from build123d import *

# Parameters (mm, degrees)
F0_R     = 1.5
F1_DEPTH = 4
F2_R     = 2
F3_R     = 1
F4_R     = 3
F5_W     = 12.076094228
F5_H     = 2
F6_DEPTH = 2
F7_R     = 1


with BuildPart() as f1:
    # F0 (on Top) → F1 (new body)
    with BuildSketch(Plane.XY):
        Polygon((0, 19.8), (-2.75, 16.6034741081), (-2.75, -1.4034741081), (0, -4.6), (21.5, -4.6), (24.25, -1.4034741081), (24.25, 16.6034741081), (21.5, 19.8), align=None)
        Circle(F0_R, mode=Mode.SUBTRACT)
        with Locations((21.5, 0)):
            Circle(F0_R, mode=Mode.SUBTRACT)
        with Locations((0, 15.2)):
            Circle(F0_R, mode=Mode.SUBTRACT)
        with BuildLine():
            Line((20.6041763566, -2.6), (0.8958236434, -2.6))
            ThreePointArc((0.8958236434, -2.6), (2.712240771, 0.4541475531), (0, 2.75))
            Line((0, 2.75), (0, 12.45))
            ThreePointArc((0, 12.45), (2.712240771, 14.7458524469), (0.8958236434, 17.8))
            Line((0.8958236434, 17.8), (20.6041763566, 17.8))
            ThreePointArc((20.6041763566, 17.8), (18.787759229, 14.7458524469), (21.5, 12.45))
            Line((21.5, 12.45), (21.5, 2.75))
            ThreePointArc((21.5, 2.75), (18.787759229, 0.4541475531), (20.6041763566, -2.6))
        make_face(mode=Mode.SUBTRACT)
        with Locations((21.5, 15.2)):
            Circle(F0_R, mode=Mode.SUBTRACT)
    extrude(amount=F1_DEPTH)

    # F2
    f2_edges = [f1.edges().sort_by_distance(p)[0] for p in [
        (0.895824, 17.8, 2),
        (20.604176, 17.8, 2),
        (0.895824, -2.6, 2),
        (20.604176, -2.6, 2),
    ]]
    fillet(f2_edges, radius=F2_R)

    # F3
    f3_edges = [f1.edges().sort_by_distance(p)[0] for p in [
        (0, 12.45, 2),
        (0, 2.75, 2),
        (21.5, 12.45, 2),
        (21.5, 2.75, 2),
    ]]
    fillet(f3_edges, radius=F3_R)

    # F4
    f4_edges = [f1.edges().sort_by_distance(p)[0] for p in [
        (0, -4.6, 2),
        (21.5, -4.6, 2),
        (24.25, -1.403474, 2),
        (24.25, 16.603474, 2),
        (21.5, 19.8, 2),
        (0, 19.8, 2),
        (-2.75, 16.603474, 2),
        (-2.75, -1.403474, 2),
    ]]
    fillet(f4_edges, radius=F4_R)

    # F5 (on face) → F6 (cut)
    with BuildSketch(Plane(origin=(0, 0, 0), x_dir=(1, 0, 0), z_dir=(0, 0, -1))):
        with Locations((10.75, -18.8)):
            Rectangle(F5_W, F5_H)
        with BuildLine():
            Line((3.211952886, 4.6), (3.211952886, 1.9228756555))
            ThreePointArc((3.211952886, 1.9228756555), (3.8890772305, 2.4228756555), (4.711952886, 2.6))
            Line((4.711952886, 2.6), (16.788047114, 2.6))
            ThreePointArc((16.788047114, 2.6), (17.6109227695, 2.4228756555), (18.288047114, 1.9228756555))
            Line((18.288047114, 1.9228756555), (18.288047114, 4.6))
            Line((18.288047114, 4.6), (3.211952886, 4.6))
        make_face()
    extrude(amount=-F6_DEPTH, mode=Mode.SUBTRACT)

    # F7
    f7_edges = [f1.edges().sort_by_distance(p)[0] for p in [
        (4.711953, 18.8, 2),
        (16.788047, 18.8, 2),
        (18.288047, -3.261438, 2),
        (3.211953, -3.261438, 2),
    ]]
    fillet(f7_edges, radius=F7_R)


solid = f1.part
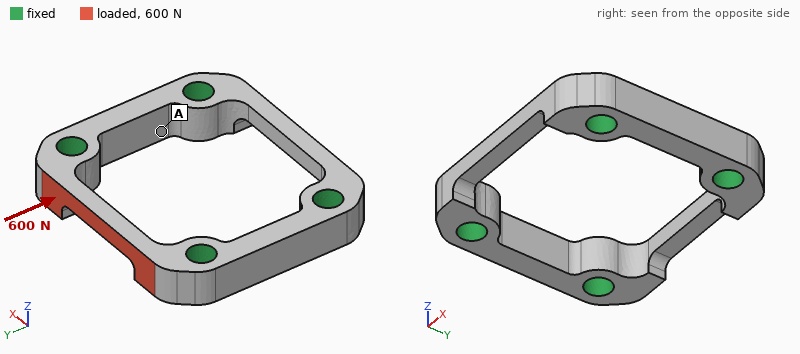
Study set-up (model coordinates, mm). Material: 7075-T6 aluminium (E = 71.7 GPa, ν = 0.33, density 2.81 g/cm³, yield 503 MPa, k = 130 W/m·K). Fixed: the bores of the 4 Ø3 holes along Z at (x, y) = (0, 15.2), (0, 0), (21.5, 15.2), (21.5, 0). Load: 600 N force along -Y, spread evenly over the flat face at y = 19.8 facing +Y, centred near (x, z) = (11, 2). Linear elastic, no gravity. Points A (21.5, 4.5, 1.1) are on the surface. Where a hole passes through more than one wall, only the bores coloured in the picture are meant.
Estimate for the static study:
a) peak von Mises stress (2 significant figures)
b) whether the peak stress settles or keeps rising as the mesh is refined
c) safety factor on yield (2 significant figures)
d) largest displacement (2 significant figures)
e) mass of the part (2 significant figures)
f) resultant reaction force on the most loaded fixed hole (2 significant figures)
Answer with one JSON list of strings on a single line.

["240 MPa", "settles", "2.1", "47 µm", "2.3 g", "330 N"]
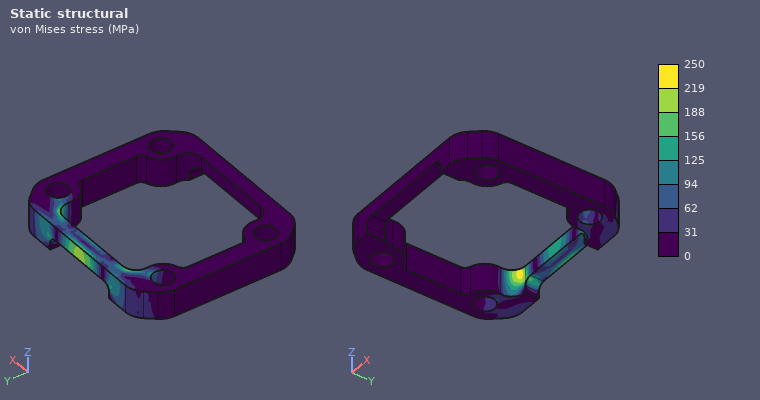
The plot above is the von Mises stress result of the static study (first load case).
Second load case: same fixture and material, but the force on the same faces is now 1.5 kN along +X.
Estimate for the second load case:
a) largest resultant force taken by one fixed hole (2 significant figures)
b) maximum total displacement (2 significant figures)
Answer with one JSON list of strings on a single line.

["760 N", "18 µm"]
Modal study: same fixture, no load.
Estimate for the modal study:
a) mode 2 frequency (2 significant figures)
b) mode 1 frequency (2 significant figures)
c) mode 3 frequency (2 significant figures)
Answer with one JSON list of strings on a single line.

["37 kHz", "35 kHz", "39 kHz"]
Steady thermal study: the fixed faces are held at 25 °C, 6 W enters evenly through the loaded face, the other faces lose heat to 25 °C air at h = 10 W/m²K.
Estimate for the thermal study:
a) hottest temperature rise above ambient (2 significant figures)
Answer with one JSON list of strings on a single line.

["17 K"]
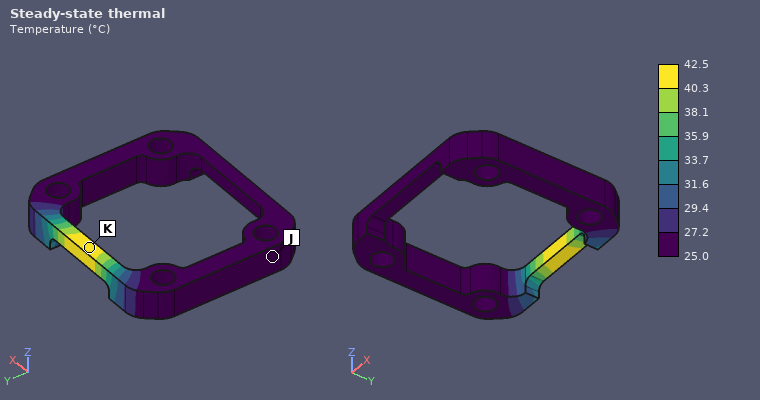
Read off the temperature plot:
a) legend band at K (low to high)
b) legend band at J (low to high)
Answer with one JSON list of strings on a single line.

["40.3 to 42.5 °C", "25.0 to 27.2 °C"]
